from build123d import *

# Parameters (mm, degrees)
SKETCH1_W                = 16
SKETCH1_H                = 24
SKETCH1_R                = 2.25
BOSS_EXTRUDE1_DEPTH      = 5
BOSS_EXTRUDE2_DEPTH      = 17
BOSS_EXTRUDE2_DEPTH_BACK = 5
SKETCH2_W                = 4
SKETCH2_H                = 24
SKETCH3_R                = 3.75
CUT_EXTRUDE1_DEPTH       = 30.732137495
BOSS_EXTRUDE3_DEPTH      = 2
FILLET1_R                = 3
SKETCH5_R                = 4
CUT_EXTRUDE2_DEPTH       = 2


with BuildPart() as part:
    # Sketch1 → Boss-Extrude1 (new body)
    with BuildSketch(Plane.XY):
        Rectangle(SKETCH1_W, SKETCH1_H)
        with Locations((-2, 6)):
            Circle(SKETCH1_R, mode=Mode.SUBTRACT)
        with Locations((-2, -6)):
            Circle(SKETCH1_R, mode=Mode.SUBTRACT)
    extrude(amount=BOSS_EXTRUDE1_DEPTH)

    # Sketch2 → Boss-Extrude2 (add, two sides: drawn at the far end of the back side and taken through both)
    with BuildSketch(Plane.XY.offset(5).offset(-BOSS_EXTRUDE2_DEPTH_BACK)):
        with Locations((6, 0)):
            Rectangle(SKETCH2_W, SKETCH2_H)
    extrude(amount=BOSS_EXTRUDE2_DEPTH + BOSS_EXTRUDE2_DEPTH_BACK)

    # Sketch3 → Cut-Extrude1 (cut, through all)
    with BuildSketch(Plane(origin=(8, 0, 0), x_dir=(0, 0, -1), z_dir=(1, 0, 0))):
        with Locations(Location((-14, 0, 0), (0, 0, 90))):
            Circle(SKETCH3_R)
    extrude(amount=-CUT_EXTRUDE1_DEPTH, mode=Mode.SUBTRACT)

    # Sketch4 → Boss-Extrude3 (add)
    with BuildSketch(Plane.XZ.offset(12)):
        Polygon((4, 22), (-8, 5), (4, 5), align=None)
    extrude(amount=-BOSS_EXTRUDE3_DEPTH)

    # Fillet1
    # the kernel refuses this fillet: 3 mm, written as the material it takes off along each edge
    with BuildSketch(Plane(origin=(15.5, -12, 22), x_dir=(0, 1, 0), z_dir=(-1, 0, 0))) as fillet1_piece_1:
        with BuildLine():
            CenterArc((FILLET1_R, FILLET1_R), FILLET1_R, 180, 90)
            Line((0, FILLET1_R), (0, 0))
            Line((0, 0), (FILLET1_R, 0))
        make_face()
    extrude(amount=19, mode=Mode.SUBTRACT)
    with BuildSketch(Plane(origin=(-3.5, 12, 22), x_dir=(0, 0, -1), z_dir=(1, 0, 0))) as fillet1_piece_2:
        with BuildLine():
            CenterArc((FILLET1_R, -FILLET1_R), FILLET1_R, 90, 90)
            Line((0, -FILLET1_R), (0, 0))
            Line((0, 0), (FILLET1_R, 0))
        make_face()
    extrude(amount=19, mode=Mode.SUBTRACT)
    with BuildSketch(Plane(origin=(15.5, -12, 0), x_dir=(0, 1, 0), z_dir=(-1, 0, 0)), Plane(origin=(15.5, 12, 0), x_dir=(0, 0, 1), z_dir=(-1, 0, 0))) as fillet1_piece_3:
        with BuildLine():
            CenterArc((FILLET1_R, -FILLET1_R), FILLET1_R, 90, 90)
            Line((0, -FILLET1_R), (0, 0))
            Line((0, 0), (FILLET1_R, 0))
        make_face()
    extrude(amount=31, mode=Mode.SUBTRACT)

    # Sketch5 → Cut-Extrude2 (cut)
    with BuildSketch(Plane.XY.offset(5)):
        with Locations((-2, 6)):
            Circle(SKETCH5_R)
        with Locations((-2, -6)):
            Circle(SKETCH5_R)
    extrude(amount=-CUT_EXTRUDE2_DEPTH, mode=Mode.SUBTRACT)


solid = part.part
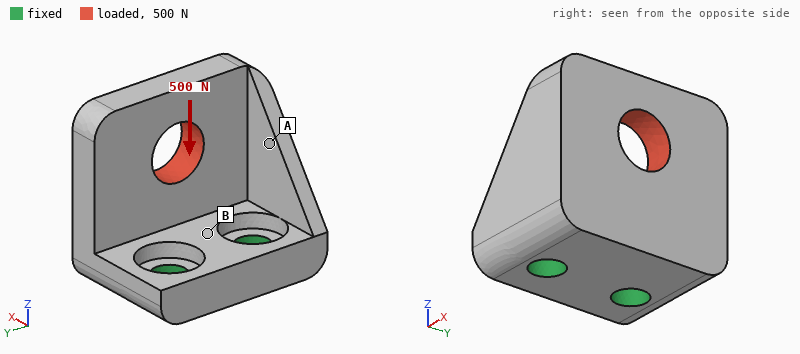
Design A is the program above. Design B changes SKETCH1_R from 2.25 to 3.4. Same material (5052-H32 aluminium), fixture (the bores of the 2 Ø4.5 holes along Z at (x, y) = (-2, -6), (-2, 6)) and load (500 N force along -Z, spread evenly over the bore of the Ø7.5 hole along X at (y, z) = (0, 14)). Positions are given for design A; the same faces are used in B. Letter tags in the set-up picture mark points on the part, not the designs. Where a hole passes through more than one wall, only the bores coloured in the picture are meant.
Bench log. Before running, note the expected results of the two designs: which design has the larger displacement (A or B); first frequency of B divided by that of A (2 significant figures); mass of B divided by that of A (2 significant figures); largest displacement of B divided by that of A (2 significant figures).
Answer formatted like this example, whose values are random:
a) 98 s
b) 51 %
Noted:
a) A
b) 1.2
c) 0.96
d) 0.58
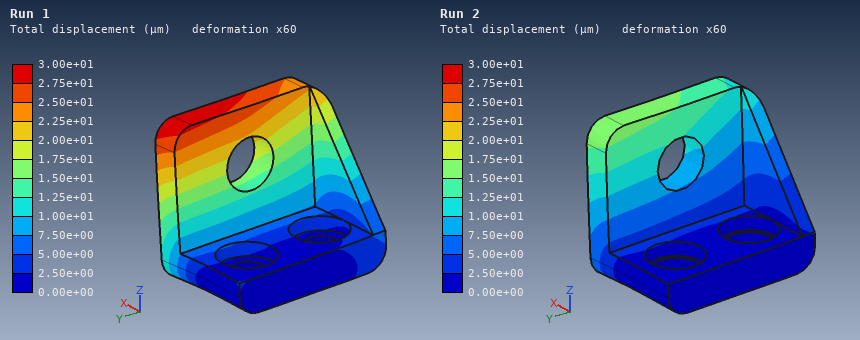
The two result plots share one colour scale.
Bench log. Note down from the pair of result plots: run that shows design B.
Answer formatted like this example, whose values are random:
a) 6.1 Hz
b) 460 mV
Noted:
a) Run 2
